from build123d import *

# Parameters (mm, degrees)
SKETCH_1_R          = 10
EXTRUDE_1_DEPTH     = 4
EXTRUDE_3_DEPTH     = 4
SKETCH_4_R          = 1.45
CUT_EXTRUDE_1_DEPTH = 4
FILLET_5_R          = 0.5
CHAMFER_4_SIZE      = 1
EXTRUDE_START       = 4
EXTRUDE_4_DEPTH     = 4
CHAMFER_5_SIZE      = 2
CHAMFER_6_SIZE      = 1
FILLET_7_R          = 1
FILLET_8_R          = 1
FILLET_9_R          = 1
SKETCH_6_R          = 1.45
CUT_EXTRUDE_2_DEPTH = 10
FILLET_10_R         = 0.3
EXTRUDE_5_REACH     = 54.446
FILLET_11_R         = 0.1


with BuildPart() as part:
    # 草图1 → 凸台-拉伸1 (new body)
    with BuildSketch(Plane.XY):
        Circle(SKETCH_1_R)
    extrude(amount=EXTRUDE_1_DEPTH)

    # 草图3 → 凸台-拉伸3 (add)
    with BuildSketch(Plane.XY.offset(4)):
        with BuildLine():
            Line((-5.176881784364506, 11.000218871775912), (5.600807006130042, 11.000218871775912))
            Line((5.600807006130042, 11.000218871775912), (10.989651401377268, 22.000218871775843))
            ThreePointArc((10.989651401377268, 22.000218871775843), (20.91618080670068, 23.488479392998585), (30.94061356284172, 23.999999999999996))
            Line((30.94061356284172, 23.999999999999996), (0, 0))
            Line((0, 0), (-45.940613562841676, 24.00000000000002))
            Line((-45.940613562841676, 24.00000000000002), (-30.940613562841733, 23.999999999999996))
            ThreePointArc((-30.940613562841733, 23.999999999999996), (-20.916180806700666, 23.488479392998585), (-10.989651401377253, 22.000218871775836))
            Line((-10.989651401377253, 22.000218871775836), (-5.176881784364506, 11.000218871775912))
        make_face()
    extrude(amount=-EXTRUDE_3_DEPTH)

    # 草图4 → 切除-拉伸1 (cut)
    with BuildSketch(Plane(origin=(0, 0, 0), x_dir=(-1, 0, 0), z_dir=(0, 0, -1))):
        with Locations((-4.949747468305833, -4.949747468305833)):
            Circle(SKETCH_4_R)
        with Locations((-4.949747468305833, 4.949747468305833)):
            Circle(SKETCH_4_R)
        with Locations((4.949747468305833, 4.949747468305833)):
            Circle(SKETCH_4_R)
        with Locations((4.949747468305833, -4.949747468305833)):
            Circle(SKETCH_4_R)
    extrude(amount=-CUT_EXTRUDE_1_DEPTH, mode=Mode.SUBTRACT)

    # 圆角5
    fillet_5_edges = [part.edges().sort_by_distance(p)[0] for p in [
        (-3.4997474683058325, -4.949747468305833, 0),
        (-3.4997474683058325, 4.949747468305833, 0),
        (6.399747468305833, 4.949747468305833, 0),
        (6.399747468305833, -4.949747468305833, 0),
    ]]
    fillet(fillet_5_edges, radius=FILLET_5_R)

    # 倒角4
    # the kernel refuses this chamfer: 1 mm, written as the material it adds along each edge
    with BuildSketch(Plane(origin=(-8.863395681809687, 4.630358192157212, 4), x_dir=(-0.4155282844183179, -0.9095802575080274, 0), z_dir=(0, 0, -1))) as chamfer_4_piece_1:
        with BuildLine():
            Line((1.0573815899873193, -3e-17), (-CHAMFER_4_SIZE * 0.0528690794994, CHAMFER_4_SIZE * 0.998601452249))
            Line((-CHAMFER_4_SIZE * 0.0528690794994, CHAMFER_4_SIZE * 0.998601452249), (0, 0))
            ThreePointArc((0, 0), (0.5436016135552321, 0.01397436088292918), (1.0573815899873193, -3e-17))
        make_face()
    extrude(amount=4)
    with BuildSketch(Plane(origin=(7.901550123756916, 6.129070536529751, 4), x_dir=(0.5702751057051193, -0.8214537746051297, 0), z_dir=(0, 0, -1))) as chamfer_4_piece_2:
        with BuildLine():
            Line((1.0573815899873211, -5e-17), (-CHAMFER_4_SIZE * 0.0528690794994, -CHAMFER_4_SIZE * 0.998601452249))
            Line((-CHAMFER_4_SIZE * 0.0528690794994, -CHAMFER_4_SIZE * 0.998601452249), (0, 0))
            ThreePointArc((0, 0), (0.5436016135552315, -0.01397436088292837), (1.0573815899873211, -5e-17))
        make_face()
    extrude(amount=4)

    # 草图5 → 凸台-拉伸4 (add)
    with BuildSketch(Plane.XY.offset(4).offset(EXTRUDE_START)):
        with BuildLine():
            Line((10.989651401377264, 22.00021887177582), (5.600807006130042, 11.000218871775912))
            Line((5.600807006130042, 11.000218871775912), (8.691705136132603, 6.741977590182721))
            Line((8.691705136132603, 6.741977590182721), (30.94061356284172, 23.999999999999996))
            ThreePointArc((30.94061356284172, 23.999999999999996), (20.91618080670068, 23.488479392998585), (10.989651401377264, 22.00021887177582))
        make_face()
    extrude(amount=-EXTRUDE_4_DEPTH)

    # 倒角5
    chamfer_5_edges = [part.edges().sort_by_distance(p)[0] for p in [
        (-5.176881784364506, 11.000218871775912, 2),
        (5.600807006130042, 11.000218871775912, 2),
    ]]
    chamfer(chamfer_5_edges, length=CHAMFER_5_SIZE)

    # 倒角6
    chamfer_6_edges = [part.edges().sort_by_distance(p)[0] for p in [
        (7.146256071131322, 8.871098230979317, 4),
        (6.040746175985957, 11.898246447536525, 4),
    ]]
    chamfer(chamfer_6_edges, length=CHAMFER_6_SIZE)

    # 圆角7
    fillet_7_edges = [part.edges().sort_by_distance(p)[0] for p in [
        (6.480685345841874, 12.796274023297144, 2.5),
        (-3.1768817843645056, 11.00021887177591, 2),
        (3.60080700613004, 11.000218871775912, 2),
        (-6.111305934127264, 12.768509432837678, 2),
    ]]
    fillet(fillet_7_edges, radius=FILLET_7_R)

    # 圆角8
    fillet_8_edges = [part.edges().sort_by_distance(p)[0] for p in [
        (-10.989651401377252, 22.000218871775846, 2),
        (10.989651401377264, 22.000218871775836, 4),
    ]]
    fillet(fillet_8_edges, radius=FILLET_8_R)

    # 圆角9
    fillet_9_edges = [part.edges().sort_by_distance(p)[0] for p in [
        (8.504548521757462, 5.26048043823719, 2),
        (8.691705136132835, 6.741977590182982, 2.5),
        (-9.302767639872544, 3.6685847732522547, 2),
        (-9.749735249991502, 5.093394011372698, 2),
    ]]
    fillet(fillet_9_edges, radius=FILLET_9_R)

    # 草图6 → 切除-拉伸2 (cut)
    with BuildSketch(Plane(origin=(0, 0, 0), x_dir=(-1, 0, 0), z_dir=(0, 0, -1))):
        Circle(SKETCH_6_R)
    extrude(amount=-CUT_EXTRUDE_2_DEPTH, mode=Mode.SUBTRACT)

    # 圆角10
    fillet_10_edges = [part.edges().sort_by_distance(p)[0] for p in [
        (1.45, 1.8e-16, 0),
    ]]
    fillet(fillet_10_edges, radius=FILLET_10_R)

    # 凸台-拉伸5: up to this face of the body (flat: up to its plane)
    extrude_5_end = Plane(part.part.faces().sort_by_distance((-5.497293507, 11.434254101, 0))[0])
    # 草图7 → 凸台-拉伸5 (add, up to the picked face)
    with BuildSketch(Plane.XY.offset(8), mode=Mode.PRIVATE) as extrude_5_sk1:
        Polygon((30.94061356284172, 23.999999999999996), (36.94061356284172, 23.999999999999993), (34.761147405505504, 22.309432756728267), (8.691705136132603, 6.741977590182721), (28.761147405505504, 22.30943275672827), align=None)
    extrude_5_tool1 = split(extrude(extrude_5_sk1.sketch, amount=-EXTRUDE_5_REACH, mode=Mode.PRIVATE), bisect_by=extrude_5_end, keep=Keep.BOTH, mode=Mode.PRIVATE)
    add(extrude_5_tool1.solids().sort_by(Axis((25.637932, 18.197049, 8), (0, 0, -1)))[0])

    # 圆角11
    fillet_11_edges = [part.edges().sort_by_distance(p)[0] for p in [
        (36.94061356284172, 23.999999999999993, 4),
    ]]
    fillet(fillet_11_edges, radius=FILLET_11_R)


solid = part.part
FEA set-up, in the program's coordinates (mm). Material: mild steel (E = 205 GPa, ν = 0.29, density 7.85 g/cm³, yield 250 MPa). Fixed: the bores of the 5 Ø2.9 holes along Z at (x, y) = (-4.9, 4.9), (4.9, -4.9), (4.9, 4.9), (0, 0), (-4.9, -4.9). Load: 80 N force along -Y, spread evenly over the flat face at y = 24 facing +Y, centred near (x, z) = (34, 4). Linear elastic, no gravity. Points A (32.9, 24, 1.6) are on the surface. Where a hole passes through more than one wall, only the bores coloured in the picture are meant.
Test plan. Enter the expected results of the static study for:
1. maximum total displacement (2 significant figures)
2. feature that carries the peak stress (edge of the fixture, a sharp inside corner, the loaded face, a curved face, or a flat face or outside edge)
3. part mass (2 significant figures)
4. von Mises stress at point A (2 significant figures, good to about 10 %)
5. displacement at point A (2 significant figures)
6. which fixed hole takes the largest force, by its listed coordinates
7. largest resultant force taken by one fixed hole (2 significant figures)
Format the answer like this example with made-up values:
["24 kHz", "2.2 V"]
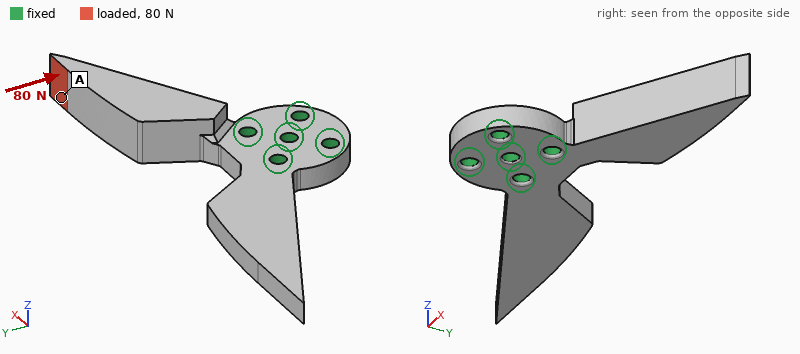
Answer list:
["31 µm", "a curved face", "36 g", "11 MPa", "26 µm", "(4.9, 4.9)", "250 N"]
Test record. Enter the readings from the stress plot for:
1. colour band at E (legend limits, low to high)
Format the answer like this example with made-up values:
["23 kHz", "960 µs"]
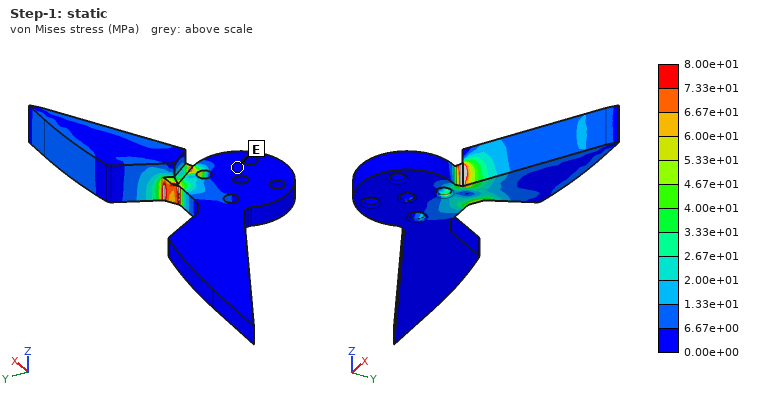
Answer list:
["0.00e+00 to 6.67e+00 MPa"]
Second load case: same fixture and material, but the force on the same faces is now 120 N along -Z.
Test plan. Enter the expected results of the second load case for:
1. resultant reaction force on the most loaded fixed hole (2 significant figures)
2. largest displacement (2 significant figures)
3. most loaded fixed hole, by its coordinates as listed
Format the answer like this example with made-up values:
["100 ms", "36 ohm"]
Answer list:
["310 N", "0.10 mm", "(4.9, 4.9)"]
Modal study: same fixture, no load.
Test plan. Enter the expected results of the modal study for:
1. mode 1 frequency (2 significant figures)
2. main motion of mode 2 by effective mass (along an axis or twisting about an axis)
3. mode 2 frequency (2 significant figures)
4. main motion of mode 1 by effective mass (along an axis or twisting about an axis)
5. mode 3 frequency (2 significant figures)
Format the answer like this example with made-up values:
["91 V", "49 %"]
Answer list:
["2400 Hz", "along Z", "2800 Hz", "along Z", "4200 Hz"]
